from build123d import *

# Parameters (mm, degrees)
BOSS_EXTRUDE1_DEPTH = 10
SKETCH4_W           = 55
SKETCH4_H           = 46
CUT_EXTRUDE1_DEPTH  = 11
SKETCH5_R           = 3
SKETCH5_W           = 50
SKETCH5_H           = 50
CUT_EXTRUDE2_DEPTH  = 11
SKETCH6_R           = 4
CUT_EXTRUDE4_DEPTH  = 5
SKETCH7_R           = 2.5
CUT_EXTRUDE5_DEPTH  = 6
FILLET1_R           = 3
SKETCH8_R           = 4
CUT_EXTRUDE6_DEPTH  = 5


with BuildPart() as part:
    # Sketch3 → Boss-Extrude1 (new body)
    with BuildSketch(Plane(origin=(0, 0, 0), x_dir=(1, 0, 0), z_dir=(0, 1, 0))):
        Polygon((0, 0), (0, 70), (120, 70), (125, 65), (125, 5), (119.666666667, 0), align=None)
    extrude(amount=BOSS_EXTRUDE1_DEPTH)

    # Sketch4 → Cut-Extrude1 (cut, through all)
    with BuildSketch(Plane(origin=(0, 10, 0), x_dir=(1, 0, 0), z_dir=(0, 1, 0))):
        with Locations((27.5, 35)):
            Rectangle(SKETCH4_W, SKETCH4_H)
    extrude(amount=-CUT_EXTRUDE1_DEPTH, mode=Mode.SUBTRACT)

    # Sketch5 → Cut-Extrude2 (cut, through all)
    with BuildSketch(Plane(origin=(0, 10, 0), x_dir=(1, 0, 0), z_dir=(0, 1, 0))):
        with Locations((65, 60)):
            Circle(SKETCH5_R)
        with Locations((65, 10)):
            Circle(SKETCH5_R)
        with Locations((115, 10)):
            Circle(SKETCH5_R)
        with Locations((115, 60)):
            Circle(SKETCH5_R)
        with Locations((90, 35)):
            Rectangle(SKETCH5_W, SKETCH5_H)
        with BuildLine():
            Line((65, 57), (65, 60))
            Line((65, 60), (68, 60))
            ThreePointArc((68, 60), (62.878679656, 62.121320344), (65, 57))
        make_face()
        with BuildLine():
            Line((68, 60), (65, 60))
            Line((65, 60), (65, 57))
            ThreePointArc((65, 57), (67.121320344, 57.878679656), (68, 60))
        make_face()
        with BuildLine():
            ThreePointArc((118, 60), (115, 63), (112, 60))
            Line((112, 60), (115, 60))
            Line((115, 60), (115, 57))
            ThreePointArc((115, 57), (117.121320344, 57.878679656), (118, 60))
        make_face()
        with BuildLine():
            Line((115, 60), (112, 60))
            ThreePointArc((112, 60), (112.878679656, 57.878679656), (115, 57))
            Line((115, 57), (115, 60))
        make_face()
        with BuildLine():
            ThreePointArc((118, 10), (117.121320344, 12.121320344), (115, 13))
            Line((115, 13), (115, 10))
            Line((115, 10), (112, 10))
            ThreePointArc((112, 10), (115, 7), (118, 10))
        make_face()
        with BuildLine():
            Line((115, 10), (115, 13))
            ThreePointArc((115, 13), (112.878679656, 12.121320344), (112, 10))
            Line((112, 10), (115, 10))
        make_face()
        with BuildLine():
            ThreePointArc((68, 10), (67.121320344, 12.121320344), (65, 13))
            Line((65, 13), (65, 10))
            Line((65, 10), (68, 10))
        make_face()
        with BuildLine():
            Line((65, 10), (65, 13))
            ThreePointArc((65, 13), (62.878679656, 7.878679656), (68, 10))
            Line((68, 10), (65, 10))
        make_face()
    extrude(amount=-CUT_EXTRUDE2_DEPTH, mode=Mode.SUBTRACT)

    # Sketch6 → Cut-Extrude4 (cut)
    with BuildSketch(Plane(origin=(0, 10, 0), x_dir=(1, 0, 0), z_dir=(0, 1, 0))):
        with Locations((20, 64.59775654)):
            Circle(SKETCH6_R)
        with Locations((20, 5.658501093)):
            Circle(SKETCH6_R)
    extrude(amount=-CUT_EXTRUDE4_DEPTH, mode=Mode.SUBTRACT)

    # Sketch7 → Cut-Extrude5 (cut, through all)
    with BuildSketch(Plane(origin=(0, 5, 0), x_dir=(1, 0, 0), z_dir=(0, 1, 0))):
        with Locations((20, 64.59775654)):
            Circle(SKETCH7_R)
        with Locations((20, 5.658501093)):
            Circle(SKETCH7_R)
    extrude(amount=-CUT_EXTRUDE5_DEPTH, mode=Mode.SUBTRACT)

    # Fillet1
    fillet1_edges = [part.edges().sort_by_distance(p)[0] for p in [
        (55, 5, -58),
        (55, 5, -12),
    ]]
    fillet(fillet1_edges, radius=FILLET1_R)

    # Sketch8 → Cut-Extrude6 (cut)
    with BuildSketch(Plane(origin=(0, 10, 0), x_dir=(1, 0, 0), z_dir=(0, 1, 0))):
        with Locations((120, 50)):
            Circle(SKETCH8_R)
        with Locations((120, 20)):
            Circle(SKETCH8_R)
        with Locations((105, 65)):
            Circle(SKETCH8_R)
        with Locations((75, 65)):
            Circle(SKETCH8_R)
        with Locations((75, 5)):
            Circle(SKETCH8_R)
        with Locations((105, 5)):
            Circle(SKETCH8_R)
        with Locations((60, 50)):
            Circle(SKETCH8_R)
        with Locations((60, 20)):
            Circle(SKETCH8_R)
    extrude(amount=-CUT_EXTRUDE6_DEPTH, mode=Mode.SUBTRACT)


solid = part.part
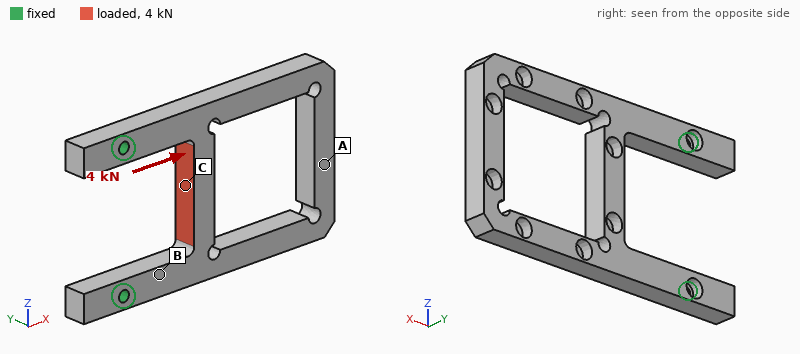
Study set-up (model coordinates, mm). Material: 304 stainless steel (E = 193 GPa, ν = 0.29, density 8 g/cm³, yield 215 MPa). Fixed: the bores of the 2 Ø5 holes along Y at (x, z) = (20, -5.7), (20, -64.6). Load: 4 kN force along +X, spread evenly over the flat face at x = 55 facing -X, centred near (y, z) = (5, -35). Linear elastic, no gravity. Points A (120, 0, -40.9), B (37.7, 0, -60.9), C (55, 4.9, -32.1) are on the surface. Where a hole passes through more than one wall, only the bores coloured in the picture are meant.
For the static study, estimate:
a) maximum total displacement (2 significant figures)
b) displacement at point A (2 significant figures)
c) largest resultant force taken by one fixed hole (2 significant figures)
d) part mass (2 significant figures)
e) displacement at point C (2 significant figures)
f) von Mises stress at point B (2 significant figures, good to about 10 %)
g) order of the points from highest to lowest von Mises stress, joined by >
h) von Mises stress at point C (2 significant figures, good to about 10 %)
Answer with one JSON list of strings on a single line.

["47 µm", "35 µm", "2.1 kN", "270 g", "37 µm", "32 MPa", "C > B > A", "85 MPa"]
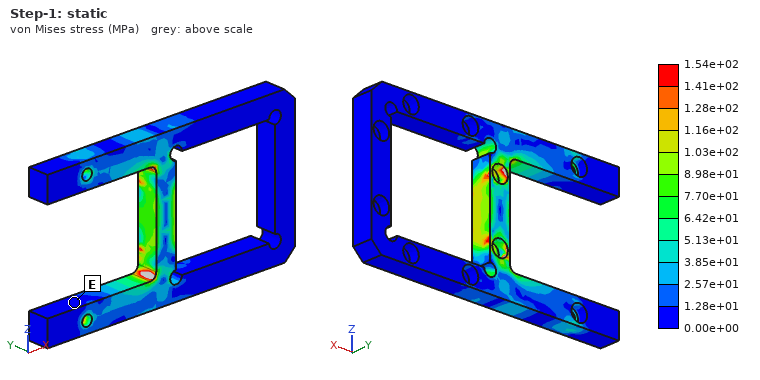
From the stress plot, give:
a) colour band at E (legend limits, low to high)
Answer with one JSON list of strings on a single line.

["0.00e+00 to 1.28e+01 MPa"]
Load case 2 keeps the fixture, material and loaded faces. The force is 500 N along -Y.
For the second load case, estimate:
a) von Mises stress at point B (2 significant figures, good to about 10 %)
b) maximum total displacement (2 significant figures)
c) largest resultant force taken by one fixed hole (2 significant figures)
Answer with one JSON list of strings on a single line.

["23 MPa", "0.12 mm", "250 N"]
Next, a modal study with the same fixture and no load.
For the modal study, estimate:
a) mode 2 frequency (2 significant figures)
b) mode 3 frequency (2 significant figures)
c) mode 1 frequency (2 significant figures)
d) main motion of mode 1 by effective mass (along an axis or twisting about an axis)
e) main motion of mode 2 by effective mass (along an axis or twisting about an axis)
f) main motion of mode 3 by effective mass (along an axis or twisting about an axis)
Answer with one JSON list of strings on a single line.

["1000 Hz", "1300 Hz", "500 Hz", "along Y", "along Z", "twisting about X"]
